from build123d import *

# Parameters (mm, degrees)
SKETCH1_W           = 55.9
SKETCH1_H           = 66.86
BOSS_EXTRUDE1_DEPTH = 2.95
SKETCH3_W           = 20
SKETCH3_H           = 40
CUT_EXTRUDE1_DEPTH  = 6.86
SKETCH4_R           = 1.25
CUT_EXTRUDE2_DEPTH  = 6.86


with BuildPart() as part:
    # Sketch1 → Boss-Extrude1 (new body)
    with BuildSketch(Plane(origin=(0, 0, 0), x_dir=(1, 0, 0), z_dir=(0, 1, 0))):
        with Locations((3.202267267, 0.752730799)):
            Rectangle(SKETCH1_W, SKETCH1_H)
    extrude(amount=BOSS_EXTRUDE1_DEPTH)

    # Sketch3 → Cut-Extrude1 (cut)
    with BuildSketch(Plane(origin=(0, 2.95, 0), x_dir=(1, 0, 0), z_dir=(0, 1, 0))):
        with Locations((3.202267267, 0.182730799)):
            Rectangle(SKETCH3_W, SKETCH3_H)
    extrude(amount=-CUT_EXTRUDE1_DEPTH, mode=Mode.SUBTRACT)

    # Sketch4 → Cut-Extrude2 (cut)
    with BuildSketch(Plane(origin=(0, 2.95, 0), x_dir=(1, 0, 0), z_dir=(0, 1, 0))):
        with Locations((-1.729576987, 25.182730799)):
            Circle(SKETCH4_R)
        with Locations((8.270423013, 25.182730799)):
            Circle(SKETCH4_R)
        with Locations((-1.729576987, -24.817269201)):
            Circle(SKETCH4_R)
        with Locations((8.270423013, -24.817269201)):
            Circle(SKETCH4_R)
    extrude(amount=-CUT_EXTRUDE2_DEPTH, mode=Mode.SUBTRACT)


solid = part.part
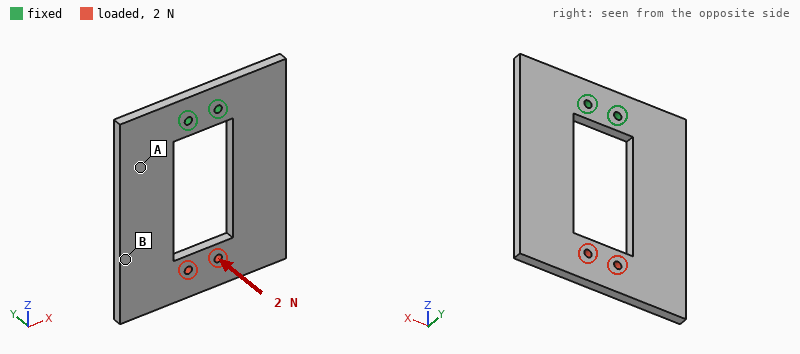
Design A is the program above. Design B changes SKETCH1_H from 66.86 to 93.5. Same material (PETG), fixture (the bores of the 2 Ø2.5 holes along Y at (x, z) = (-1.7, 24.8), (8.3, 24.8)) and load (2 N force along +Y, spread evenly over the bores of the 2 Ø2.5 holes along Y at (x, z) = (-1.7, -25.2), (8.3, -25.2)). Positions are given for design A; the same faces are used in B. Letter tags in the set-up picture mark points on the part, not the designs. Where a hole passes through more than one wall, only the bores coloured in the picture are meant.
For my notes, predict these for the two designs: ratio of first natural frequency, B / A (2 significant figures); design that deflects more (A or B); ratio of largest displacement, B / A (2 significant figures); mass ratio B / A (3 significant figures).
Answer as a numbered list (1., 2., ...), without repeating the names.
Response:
1. 0.69
2. B
3. 1.2
4. 1.51
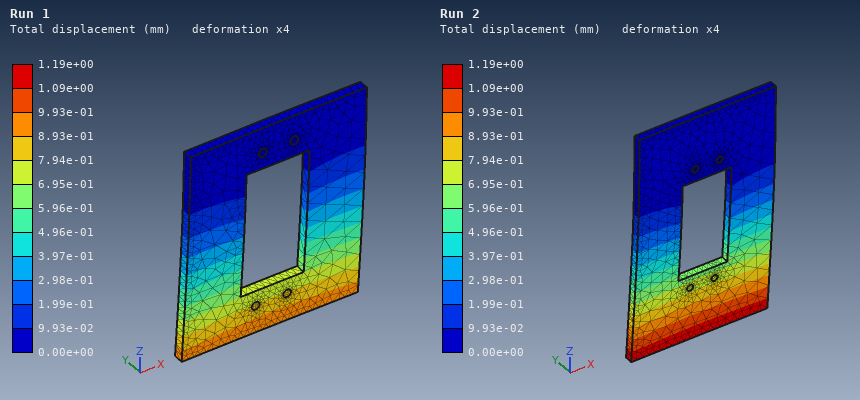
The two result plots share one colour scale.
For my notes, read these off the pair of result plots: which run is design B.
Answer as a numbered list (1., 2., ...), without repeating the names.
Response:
1. Run 2
